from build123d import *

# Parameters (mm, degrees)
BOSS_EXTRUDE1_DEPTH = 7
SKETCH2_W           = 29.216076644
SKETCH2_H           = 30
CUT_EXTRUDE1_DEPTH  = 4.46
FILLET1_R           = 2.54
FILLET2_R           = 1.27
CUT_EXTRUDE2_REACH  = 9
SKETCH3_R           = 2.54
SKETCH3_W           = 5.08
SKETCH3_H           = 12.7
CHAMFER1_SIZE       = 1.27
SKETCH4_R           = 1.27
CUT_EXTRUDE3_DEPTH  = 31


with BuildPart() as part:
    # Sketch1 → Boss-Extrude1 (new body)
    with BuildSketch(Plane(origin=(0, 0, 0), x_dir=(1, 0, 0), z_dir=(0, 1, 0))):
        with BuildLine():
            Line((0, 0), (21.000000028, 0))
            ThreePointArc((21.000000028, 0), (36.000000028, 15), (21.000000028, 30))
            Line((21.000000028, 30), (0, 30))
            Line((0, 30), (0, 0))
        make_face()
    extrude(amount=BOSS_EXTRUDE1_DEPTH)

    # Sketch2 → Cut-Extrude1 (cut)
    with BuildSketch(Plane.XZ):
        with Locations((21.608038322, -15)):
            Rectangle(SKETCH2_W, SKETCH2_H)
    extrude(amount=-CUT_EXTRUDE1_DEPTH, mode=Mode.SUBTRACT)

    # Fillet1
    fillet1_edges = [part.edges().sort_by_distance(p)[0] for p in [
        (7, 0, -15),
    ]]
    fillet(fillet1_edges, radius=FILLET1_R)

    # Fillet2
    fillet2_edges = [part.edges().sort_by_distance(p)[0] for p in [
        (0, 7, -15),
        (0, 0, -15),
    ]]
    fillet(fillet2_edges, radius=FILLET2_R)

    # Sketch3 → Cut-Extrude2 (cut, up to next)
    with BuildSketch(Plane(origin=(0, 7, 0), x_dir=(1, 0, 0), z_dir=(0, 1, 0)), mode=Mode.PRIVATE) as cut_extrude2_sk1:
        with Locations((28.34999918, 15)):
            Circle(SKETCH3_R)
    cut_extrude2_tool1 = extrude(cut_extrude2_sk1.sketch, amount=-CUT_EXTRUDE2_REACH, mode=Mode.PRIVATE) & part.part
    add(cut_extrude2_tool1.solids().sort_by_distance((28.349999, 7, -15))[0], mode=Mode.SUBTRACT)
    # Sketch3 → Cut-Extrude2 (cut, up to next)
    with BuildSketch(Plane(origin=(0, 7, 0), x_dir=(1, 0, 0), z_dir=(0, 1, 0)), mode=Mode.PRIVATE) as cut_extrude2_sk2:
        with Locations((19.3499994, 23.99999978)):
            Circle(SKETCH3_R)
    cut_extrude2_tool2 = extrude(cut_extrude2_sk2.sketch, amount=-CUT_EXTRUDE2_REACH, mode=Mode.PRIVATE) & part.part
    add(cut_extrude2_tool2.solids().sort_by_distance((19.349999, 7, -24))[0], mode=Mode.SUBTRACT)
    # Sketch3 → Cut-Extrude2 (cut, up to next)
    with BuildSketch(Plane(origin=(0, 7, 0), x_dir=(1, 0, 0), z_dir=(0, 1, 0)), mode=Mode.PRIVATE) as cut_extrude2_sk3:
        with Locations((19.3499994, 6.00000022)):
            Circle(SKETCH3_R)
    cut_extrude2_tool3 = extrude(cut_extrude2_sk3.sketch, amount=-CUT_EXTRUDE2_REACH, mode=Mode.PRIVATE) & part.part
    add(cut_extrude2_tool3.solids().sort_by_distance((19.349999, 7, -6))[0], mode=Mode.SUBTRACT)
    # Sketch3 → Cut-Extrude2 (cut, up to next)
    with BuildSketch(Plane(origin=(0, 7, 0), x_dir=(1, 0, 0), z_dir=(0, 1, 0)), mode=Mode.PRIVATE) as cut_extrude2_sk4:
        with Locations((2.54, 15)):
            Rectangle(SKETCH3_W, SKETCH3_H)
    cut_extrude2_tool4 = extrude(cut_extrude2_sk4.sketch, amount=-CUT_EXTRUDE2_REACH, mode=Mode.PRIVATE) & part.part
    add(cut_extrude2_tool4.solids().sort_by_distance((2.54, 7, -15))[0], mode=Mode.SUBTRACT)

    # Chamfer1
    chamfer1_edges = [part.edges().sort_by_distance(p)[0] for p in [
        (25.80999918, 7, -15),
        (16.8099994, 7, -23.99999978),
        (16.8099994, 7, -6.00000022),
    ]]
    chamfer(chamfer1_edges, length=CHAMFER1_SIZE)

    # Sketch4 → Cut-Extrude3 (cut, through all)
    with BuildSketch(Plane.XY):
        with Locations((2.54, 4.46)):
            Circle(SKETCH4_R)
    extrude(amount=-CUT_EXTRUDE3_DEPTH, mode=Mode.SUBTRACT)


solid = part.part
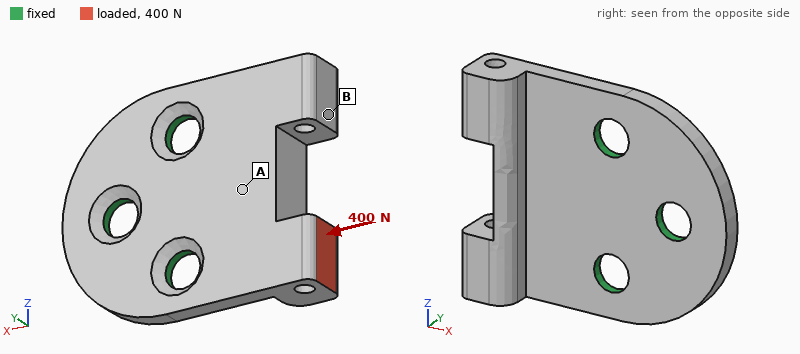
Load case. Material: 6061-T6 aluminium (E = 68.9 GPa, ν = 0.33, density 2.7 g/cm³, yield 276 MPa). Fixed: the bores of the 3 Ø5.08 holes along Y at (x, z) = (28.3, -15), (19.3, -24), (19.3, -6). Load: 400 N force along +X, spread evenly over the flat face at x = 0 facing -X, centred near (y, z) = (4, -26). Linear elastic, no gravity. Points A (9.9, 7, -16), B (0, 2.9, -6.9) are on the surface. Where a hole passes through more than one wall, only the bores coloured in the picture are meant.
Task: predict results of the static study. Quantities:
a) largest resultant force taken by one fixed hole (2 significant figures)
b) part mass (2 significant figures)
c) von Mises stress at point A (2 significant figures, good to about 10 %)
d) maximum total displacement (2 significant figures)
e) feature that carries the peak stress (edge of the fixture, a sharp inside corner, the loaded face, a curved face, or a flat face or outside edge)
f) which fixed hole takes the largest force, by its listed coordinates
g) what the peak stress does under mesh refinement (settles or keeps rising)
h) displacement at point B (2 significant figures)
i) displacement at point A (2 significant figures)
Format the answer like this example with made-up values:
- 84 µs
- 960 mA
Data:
- 400 N
- 7.1 g
- 27 MPa
- 87 µm
- edge of the fixture
- (19.3, -24)
- keeps rising
- 31 µm
- 15 µm
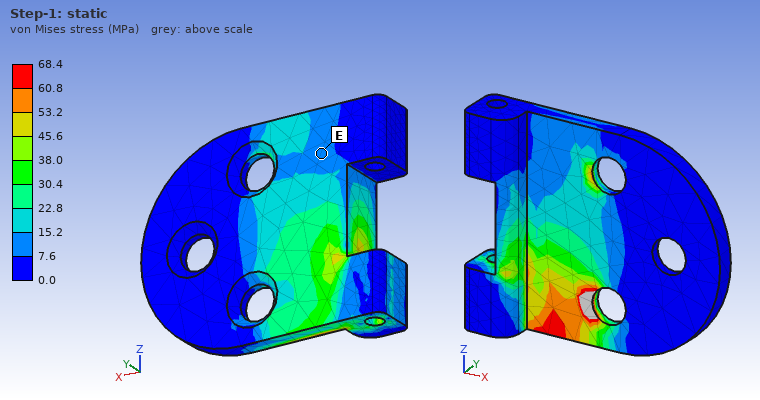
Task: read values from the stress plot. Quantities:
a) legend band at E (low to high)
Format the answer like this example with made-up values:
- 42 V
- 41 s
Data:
- 7.6 to 15.2 MPa
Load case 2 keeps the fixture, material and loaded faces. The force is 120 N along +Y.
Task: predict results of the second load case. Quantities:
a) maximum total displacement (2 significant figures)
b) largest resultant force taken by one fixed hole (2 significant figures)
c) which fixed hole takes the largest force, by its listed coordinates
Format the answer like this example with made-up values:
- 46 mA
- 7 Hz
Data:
- 0.17 mm
- 170 N
- (19.3, -24)
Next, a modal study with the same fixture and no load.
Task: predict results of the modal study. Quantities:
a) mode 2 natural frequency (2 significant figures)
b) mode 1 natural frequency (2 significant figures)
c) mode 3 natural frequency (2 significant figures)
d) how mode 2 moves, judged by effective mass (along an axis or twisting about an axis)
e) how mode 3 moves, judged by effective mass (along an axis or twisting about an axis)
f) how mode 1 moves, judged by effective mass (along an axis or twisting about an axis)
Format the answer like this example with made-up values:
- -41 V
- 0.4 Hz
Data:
- 6400 Hz
- 4400 Hz
- 20 kHz
- twisting about X
- along Z
- along Y
